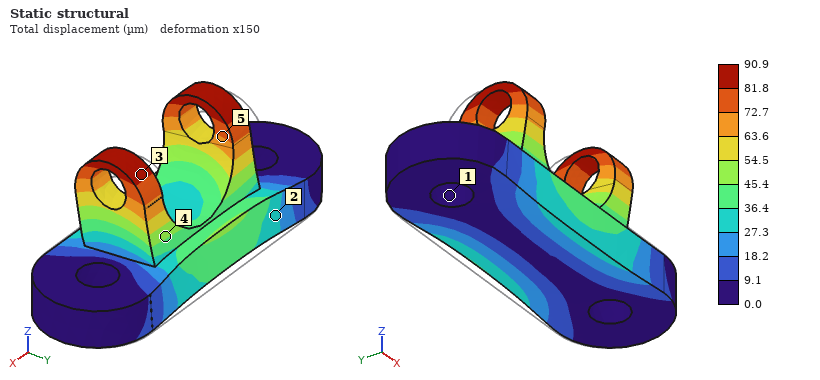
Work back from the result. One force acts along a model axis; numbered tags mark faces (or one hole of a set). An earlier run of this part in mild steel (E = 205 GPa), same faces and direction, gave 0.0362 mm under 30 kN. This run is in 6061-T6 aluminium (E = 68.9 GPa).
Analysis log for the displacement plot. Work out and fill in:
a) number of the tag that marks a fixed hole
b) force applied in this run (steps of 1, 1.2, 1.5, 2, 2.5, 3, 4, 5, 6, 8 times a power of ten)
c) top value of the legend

1
25 kN
90.9 µm
